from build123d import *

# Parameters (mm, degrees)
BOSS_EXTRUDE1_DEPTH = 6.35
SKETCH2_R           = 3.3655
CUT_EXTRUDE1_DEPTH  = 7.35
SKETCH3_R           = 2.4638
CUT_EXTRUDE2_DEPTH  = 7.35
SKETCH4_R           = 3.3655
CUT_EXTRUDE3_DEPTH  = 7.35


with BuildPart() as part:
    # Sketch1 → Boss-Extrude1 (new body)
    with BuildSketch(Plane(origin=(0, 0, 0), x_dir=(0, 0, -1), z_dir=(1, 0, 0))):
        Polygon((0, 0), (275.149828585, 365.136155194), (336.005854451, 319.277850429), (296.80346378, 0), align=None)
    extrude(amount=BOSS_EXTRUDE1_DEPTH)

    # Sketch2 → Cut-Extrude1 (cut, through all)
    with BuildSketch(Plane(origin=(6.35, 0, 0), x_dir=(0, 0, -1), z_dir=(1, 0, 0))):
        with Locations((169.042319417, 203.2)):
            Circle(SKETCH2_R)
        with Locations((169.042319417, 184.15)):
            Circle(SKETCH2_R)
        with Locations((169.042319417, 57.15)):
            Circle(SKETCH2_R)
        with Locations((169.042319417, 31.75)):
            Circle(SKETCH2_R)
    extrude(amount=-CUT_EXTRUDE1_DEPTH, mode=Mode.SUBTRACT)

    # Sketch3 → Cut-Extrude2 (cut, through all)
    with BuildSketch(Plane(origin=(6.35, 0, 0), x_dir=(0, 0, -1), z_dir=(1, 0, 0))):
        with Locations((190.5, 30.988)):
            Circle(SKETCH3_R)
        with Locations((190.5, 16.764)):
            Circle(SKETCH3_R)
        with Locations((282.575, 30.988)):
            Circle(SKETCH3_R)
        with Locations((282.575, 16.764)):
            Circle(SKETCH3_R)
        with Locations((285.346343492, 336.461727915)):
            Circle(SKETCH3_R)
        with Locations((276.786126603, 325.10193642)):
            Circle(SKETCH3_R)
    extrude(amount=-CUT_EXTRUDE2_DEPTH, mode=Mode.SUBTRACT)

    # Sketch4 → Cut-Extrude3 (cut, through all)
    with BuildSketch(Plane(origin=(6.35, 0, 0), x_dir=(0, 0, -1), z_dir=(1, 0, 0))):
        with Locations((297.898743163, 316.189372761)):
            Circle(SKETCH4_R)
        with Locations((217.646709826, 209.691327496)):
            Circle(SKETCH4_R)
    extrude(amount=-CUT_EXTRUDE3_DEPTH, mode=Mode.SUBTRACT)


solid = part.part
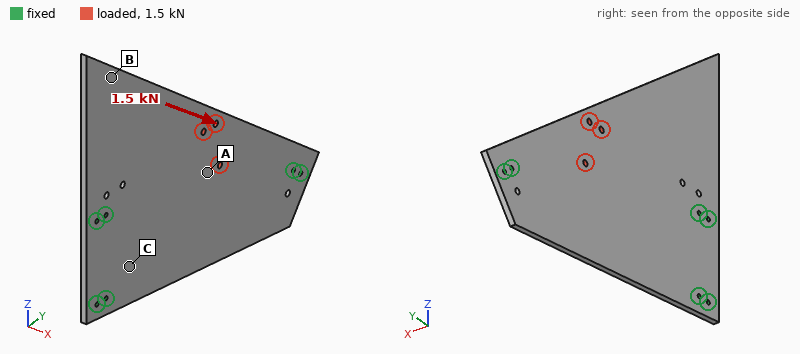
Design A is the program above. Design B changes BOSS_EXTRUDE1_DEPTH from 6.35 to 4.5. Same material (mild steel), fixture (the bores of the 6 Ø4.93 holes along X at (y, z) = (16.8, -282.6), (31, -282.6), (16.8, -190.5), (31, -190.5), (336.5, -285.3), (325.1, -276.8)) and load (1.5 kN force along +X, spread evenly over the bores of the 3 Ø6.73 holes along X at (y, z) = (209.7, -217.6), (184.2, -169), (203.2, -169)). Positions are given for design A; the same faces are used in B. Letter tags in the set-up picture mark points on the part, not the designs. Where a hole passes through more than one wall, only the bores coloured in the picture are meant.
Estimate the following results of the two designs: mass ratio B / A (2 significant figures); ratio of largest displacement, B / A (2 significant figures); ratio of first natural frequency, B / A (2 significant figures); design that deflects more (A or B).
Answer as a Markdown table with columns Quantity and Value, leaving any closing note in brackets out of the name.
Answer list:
| Quantity | Value |
|---|---|
| mass ratio B / A | 0.71 |
| ratio of largest displacement, B / A | 2.8 |
| ratio of first natural frequency, B / A | 0.72 |
| design that deflects more | B |
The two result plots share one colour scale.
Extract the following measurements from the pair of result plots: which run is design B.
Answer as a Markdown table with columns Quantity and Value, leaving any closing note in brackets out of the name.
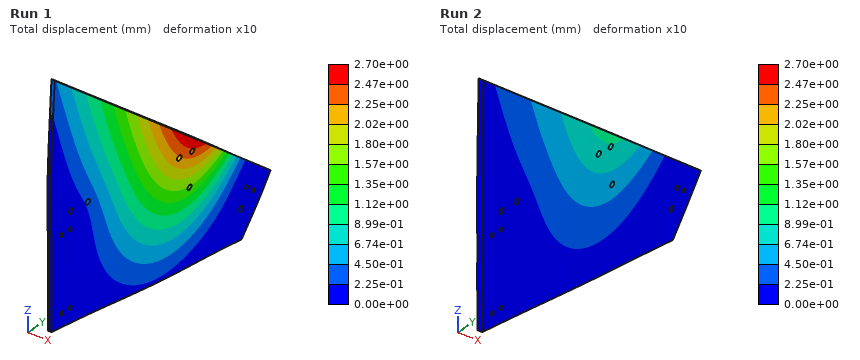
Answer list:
| Quantity | Value |
|---|---|
| which run is design B | Run 1 |
